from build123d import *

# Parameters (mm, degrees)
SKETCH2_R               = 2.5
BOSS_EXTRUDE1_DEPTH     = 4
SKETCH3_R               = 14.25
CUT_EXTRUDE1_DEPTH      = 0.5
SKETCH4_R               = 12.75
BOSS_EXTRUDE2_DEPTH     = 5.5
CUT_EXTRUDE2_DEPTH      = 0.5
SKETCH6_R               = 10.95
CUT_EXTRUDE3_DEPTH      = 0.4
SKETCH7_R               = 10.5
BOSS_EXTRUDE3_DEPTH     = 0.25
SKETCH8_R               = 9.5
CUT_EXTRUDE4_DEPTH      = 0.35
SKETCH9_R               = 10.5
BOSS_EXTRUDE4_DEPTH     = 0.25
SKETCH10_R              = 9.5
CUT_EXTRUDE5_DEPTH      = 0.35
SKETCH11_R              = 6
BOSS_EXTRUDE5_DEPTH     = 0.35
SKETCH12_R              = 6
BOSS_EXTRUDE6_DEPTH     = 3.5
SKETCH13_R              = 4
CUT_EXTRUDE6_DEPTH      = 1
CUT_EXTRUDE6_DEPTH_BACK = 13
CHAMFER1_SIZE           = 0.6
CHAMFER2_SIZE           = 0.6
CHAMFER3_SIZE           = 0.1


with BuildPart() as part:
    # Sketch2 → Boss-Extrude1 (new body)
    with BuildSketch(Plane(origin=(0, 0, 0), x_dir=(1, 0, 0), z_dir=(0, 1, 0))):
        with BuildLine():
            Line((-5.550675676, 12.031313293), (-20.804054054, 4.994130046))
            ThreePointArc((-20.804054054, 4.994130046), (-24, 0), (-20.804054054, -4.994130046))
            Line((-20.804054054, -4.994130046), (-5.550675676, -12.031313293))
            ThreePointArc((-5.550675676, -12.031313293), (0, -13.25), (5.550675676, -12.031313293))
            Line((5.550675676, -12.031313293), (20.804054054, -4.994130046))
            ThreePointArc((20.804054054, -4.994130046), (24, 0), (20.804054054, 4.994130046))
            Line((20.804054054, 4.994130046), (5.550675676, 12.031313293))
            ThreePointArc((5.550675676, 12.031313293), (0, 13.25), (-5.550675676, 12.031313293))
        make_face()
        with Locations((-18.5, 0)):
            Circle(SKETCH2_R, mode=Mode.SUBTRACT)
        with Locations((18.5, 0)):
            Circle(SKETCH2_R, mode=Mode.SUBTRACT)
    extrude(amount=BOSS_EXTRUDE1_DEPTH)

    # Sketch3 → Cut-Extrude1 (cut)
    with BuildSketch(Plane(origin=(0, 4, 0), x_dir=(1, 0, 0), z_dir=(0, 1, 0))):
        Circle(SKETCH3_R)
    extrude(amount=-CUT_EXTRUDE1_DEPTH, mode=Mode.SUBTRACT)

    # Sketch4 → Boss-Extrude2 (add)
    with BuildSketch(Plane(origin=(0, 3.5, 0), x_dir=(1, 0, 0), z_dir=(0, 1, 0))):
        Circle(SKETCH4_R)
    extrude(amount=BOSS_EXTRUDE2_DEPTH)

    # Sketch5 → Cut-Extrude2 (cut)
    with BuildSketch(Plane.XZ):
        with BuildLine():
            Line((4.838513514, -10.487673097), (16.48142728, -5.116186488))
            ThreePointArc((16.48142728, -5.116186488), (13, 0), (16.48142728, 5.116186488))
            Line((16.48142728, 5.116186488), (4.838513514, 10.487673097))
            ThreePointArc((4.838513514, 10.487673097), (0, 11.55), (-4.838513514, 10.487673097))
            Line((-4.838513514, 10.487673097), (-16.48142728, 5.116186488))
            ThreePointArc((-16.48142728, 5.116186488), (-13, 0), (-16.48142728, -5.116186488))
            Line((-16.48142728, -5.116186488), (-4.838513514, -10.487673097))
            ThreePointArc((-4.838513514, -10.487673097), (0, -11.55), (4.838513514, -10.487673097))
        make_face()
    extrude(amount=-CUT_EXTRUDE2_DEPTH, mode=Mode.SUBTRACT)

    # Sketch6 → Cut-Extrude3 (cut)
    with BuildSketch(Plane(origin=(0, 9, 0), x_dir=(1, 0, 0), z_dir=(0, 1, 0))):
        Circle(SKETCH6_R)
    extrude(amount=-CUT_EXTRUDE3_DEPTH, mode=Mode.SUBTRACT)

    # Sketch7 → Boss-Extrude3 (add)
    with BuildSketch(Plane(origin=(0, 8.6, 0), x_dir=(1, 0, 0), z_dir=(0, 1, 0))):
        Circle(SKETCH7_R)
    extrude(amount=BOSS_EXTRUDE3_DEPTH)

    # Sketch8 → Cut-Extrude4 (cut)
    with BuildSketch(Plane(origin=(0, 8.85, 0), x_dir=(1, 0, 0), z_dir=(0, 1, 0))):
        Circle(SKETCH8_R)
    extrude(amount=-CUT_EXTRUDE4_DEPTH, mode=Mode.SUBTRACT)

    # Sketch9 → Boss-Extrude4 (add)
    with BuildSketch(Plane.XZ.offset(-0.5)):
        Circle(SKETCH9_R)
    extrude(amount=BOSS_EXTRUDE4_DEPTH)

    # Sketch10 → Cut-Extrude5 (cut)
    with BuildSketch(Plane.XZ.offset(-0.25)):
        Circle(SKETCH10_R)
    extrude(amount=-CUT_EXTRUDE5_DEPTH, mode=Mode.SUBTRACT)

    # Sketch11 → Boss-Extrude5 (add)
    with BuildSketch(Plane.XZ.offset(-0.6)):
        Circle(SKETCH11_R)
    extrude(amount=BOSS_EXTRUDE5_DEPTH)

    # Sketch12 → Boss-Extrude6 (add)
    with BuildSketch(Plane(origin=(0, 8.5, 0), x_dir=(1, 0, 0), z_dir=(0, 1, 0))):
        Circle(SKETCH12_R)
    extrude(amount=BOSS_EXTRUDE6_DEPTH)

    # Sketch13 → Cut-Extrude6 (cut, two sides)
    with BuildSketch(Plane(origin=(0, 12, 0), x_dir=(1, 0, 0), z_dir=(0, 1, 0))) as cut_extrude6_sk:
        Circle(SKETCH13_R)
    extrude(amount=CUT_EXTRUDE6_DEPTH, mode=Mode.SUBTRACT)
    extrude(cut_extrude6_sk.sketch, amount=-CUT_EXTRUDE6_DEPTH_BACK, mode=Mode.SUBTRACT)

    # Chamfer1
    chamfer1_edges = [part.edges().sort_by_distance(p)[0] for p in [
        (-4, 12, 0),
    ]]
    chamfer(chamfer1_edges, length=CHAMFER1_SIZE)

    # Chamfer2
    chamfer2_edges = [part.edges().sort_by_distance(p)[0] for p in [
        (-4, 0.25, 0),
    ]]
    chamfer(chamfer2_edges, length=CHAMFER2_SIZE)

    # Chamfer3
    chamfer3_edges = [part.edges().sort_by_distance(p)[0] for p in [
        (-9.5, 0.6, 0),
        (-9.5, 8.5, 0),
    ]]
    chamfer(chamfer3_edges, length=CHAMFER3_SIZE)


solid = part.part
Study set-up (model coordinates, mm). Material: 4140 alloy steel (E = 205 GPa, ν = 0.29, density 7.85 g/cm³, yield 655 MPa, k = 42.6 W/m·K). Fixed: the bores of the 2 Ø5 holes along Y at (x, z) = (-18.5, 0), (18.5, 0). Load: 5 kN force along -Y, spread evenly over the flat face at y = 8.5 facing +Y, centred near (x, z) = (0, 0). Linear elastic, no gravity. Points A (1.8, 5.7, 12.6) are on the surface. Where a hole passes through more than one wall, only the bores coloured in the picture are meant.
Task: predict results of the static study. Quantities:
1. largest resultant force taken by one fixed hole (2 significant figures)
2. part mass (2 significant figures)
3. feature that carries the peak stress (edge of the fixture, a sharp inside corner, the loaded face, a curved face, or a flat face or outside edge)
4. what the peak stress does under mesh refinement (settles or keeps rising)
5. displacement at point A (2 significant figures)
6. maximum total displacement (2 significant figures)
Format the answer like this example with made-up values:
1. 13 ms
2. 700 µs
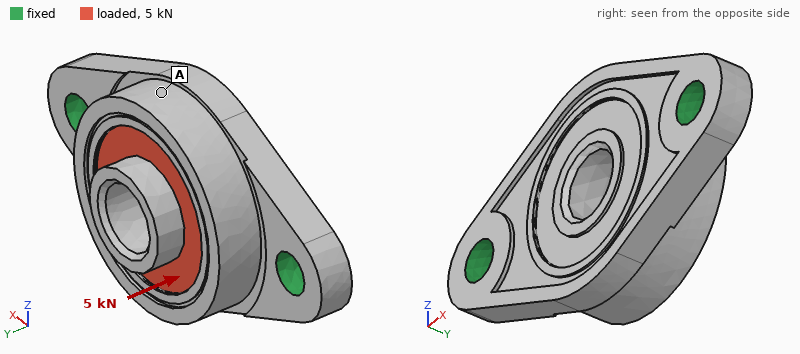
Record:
1. 3.1 kN
2. 40 g
3. edge of the fixture
4. keeps rising
5. 20 µm
6. 20 µm
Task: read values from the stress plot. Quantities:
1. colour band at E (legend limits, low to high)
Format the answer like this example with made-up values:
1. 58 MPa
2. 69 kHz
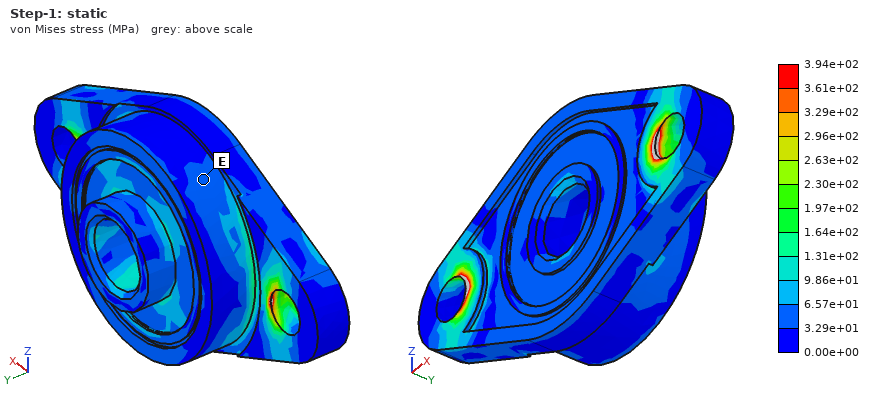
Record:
1. 3.29e+01 to 6.57e+01 MPa
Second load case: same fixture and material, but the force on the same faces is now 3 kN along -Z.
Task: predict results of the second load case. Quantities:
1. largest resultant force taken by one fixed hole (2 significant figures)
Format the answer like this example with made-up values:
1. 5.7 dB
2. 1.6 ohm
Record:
1. 1.5 kN
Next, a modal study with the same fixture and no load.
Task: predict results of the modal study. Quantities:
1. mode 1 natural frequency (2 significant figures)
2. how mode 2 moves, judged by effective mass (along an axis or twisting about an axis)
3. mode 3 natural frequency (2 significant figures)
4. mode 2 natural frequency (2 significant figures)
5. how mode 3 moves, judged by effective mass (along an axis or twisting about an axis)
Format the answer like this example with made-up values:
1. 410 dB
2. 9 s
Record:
1. 9300 Hz
2. along Y
3. 26 kHz
4. 15 kHz
5. along Z
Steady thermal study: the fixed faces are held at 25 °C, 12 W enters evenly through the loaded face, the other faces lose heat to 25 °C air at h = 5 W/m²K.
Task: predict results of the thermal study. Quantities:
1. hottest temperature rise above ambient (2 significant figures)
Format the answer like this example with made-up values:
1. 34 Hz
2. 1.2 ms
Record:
1. 28 K
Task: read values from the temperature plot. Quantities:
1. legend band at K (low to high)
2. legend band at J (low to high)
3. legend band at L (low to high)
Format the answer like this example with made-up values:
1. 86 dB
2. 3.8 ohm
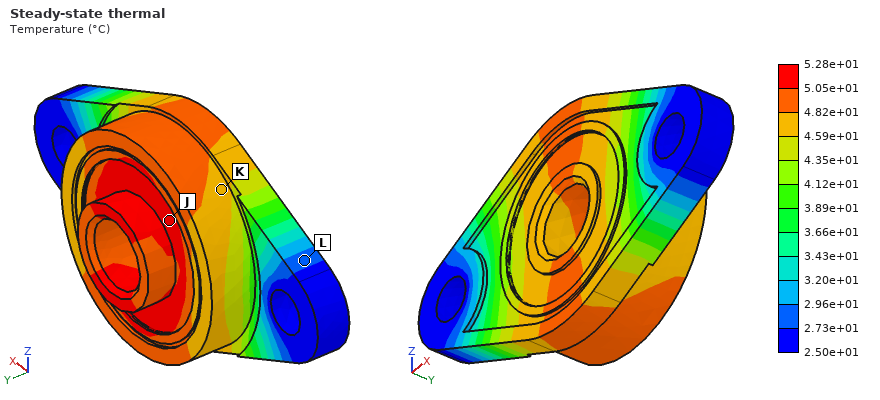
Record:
1. 4.59e+01 to 4.82e+01 °C
2. 5.05e+01 to 5.28e+01 °C
3. 2.73e+01 to 2.96e+01 °C
